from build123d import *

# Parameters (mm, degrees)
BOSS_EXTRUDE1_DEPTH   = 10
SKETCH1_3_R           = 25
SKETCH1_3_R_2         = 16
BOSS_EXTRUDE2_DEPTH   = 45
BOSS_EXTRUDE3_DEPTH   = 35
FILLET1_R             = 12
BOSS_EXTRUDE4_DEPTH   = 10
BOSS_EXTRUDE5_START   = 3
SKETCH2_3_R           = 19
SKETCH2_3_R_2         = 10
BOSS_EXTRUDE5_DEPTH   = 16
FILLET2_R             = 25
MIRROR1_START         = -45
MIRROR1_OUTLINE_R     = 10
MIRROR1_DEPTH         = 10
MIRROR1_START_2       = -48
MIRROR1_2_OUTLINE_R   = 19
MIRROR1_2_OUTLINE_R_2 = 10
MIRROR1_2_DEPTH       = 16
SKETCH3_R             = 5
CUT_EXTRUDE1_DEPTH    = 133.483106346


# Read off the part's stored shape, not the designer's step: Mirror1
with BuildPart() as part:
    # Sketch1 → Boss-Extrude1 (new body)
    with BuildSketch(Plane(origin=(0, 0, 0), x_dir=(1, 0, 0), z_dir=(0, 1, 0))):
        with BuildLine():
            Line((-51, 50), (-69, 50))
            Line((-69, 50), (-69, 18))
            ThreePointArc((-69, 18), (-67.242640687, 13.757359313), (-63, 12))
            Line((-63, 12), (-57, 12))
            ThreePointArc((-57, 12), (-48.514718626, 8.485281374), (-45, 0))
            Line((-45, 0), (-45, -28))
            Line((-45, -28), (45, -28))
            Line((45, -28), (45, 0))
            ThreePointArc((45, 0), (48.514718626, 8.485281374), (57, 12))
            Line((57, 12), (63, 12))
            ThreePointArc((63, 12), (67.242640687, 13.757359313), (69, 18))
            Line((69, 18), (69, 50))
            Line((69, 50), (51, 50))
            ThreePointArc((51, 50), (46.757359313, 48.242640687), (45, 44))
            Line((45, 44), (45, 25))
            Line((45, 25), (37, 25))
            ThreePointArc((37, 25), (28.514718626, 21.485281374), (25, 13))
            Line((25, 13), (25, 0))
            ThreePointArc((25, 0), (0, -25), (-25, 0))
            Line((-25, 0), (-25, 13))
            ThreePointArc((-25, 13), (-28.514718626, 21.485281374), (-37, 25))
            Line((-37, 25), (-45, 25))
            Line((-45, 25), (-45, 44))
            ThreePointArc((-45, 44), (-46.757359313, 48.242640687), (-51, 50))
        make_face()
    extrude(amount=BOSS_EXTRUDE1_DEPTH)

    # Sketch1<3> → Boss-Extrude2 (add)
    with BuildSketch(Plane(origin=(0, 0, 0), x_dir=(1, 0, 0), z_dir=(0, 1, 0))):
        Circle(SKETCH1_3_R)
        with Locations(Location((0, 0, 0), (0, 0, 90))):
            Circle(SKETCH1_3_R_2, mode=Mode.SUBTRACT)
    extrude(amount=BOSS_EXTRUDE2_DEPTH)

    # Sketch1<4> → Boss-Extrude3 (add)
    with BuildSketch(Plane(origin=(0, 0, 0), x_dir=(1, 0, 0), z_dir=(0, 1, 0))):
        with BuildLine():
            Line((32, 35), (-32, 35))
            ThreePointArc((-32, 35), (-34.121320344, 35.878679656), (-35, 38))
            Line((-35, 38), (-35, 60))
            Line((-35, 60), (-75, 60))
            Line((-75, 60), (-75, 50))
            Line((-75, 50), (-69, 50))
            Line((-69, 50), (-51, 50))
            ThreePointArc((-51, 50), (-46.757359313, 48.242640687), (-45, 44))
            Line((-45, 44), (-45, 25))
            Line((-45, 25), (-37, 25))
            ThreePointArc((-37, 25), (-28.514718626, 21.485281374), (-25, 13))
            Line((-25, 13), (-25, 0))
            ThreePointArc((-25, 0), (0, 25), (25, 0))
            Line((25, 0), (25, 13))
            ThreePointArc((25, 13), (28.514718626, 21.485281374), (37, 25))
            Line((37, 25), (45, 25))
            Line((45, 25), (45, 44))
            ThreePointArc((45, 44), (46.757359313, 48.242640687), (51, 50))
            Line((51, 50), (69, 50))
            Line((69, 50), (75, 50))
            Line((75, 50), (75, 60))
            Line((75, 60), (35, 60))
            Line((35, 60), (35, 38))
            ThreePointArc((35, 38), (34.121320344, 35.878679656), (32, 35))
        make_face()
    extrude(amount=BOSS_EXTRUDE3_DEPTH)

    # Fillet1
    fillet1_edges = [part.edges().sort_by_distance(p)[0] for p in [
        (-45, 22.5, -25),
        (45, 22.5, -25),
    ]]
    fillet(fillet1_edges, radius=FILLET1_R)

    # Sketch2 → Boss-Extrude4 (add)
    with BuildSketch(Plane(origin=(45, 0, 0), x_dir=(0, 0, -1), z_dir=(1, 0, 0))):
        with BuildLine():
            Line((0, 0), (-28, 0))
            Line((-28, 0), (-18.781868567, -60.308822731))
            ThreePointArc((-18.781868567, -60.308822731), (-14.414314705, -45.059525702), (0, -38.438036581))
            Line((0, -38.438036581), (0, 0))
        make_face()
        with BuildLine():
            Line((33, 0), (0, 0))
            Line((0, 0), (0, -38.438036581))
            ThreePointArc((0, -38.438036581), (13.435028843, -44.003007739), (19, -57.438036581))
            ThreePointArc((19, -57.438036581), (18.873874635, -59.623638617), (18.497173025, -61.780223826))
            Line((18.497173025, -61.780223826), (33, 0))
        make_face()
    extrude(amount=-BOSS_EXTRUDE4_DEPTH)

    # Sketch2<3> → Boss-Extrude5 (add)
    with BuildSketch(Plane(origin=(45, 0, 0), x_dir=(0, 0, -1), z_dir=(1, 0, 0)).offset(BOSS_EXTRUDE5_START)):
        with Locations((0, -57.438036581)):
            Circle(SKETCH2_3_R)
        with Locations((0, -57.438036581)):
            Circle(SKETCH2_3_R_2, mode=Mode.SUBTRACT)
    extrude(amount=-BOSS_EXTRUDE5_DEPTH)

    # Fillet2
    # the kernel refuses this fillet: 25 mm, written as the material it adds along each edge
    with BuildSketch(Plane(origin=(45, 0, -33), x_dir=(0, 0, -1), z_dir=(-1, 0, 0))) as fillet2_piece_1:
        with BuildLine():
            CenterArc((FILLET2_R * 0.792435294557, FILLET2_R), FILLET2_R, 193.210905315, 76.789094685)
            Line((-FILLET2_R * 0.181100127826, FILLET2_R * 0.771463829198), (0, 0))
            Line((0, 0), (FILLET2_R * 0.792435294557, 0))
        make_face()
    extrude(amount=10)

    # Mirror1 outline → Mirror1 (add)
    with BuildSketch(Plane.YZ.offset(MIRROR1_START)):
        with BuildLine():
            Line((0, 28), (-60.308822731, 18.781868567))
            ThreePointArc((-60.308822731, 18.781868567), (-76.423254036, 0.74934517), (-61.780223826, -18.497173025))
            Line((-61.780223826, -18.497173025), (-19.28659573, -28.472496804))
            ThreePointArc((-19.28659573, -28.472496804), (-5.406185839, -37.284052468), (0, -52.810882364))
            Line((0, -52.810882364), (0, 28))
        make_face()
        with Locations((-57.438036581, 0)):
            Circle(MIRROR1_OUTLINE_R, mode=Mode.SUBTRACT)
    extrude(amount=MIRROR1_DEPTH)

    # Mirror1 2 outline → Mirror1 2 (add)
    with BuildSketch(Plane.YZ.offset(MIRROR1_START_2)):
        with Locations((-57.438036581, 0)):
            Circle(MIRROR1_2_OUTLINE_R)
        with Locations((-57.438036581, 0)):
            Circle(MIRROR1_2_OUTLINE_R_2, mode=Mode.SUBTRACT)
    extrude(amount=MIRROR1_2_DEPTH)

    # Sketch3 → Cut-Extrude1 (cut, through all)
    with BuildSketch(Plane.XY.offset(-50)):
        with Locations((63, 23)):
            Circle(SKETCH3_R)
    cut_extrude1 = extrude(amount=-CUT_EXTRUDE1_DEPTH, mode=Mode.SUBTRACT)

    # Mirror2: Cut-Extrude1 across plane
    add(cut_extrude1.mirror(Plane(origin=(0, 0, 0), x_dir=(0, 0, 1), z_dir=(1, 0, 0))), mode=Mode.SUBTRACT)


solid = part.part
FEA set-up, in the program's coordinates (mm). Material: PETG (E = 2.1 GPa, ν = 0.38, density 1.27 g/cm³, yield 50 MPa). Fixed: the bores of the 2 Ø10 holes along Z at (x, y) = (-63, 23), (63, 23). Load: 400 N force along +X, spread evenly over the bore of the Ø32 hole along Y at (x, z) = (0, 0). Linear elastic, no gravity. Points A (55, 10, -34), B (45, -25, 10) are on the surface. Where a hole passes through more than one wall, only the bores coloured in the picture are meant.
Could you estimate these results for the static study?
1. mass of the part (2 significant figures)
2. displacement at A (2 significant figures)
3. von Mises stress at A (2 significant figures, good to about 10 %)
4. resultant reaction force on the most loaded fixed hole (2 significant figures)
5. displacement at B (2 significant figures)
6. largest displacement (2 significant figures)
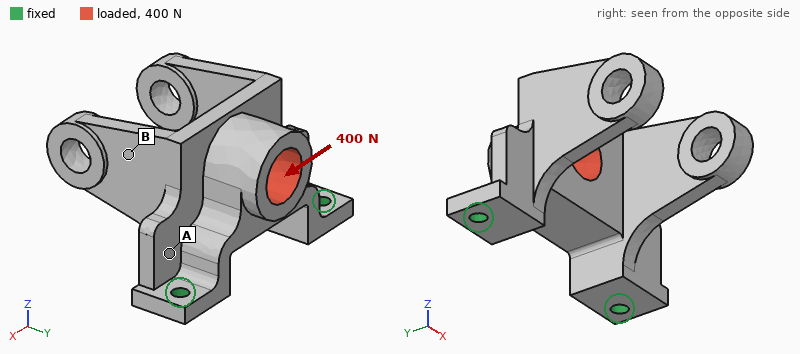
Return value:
320 g
0.045 mm
0.76 MPa
270 N
0.062 mm
0.11 mm
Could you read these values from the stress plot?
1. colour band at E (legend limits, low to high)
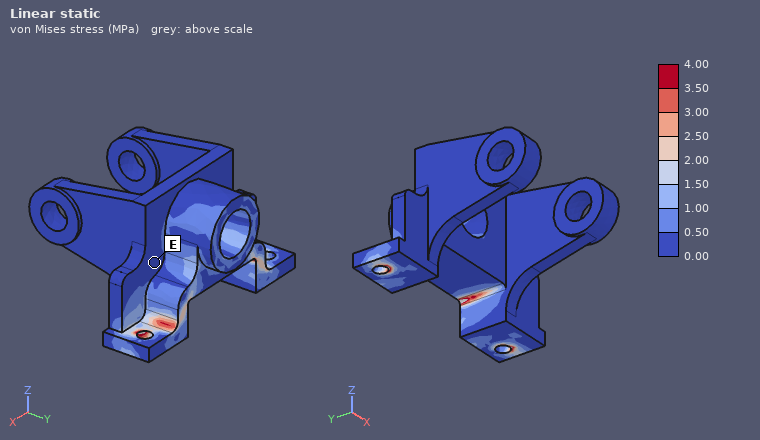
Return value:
0.00 to 0.50 MPa
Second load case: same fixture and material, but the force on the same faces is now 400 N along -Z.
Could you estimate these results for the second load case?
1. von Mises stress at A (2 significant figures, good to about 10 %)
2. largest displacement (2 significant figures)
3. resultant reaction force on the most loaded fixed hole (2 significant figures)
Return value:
0.63 MPa
0.17 mm
250 N
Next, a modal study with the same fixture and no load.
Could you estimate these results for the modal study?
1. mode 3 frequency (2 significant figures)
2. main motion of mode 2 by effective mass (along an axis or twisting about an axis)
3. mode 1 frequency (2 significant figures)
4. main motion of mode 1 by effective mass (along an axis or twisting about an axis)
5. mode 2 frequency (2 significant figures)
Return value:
320 Hz
along X
170 Hz
along Y
300 Hz
